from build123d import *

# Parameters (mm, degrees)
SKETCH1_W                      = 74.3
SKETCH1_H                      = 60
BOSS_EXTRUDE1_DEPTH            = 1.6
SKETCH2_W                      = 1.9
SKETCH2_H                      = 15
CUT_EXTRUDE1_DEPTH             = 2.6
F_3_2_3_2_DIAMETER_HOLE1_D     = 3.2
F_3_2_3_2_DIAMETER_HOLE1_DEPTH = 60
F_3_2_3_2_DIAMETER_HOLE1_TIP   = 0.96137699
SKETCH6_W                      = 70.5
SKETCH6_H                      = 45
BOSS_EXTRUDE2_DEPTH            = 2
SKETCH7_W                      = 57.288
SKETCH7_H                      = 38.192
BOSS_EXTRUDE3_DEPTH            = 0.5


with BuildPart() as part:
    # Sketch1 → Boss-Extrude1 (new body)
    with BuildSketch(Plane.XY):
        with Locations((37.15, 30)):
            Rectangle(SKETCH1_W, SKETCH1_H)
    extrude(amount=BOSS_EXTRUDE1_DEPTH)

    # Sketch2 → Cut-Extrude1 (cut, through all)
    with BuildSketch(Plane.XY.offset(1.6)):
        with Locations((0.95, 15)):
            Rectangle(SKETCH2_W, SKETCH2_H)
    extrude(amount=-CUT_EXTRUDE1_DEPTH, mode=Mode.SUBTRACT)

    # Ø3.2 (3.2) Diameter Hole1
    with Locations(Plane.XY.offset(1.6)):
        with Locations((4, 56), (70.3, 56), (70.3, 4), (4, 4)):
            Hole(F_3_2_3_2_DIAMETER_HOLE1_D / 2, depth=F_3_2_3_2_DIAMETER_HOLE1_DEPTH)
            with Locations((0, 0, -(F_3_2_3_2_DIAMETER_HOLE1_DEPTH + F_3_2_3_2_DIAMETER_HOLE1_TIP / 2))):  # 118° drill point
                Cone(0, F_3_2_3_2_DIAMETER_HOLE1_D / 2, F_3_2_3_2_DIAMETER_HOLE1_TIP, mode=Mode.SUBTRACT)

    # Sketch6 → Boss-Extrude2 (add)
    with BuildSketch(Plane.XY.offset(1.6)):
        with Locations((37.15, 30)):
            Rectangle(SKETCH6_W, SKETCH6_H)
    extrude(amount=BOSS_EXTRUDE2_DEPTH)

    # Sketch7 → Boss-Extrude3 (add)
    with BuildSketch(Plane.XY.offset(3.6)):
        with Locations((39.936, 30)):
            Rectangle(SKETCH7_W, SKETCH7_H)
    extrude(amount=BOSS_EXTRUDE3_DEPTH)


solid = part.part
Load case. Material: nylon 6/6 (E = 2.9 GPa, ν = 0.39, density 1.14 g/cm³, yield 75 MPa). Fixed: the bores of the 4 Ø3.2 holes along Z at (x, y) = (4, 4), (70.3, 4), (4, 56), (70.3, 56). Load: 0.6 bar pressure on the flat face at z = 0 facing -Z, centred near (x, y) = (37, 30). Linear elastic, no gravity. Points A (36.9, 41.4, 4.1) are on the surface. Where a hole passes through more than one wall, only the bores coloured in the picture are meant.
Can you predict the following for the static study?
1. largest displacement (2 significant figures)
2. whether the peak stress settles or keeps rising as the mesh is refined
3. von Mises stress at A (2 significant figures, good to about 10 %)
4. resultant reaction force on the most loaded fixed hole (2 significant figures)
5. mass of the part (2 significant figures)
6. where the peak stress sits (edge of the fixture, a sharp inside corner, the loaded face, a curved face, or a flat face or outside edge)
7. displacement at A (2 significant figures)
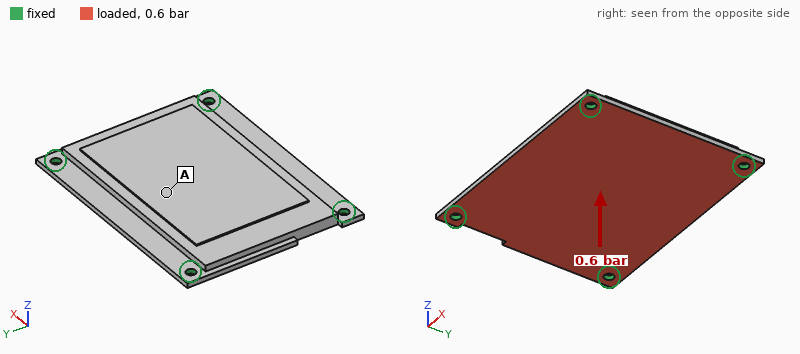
0.90 mm
keeps rising
9.8 MPa
160 N
17 g
edge of the fixture
0.76 mm
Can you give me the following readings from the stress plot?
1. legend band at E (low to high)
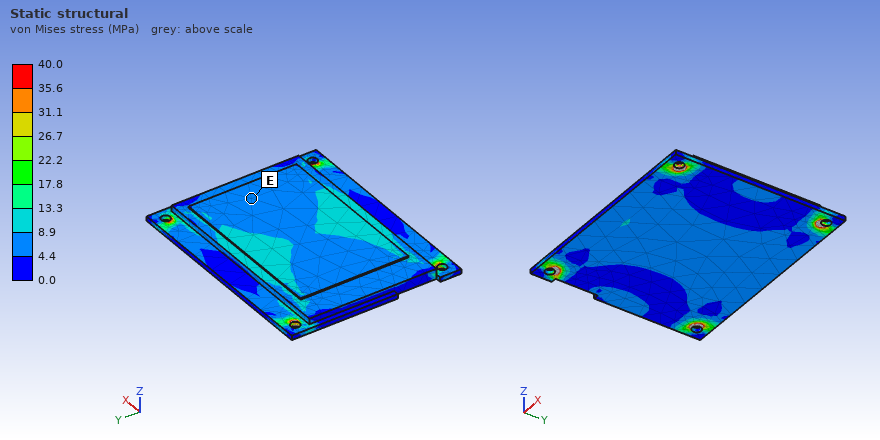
4.4 to 8.9 MPa
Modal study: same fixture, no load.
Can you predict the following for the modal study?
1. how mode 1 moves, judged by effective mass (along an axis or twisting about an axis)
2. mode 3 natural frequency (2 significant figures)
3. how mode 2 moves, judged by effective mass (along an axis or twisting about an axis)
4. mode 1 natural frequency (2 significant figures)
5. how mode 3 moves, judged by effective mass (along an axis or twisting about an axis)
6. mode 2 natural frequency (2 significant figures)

along Z
1700 Hz
twisting about X
790 Hz
twisting about Y
1300 Hz
